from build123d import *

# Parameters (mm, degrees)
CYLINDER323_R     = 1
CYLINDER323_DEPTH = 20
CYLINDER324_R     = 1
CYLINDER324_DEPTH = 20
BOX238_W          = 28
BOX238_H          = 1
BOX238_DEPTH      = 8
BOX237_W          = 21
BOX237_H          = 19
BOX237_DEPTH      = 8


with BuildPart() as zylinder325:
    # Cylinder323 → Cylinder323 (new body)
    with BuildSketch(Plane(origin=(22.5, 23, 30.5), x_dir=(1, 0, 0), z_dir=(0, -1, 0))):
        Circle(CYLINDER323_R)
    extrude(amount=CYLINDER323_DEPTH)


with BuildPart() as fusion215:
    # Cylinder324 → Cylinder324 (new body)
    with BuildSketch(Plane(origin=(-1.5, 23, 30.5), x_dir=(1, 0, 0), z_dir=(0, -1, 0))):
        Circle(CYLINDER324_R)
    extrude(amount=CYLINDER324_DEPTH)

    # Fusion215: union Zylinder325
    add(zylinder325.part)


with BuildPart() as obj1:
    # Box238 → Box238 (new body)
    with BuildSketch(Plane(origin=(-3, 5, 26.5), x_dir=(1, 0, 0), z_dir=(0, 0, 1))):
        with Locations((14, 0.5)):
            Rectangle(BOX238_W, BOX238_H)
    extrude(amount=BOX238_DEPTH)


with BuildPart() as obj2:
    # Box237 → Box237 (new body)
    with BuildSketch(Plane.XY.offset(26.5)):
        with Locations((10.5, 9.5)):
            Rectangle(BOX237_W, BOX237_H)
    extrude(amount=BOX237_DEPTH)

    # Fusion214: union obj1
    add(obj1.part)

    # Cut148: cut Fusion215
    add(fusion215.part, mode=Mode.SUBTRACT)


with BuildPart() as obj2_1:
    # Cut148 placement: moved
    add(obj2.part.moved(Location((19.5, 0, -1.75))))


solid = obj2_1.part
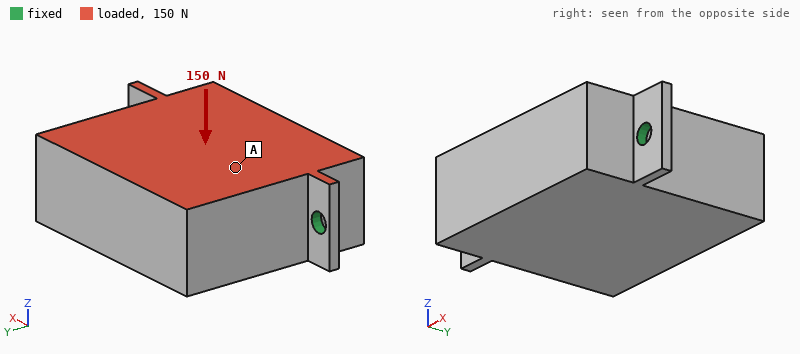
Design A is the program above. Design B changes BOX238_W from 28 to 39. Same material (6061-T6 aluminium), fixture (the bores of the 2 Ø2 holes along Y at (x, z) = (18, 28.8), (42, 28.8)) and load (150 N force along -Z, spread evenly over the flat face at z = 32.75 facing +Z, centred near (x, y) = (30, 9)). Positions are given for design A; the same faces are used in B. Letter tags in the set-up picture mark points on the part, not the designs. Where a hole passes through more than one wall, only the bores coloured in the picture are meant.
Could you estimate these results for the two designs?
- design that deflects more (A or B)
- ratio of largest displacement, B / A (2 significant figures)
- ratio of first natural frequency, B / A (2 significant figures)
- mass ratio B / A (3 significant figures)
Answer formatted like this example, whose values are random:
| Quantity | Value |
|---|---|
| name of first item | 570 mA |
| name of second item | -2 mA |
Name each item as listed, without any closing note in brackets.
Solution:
| Quantity | Value |
|---|---|
| design that deflects more | A |
| ratio of largest displacement, B / A | 0.90 |
| ratio of first natural frequency, B / A | 1.0 |
| mass ratio B / A | 1.03 |
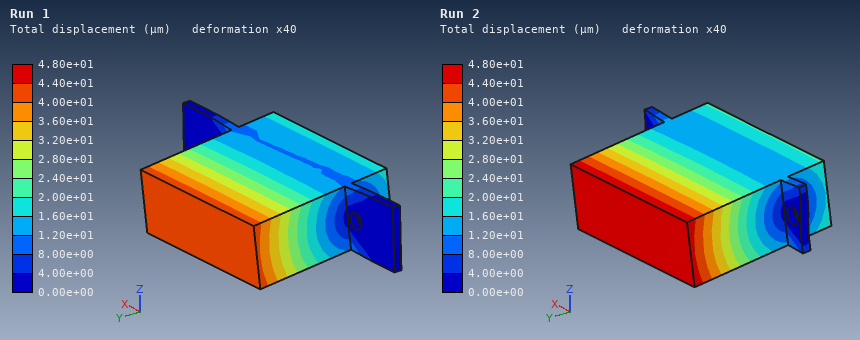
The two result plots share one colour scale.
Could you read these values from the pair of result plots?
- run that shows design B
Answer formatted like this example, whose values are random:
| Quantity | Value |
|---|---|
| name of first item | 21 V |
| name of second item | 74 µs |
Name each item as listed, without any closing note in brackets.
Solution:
| Quantity | Value |
|---|---|
| run that shows design B | Run 1 |
